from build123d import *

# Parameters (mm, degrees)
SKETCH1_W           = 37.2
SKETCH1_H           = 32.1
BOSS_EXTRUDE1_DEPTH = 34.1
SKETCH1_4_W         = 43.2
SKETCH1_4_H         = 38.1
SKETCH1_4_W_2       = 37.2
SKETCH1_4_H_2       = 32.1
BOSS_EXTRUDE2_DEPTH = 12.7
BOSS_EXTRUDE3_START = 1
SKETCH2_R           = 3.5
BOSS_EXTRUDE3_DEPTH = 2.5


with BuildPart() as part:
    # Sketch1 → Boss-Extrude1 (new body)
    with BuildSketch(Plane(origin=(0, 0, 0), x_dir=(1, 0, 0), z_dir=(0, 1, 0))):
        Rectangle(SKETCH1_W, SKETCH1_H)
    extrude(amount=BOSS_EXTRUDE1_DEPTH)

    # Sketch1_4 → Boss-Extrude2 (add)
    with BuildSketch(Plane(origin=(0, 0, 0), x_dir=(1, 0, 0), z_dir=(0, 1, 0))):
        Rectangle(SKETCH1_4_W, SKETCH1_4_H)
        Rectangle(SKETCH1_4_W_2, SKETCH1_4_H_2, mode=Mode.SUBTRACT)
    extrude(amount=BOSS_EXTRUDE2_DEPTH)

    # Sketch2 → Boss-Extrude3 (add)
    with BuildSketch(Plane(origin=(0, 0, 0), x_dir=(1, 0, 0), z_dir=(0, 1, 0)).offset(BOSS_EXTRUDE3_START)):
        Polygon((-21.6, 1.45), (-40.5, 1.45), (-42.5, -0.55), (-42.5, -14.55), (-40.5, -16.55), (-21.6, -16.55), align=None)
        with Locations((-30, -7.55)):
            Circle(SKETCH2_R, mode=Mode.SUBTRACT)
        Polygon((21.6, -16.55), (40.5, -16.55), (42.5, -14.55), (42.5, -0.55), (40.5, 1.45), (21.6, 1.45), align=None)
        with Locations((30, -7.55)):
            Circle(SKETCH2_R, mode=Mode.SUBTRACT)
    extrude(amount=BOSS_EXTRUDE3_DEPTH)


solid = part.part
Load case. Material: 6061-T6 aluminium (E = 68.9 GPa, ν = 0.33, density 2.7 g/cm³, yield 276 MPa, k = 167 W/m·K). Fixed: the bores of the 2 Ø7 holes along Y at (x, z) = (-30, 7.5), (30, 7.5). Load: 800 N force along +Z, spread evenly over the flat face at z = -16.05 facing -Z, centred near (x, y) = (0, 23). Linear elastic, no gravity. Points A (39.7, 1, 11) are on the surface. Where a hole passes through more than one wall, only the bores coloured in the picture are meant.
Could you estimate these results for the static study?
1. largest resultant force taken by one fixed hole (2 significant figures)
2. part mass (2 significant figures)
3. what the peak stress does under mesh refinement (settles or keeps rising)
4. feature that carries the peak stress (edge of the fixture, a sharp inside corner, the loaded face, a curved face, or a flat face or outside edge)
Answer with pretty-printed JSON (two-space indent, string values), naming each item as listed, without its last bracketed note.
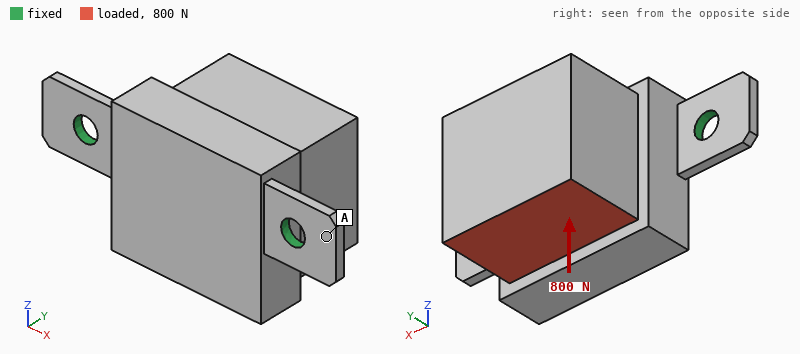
{
  "largest resultant force taken by one fixed hole": "400 N",
  "part mass": "130 g",
  "what the peak stress does under mesh refinement": "keeps rising",
  "feature that carries the peak stress": "edge of the fixture"
}
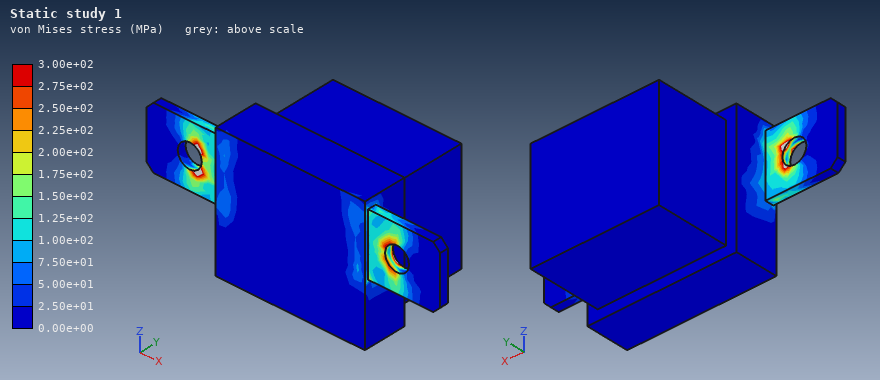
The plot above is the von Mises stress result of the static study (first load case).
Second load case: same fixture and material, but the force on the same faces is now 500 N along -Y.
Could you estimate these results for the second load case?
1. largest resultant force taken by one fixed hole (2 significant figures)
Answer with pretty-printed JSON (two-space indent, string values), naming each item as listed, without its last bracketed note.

{
  "largest resultant force taken by one fixed hole": "270 N"
}
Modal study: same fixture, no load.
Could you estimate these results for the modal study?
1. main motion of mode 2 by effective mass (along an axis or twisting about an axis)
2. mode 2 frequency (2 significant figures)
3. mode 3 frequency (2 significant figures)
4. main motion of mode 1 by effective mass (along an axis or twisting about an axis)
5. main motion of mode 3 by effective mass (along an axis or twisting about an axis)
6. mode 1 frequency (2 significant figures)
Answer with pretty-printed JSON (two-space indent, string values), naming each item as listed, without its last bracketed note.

{
  "main motion of mode 2 by effective mass": "along Y",
  "mode 2 frequency": "4000 Hz",
  "mode 3 frequency": "4400 Hz",
  "main motion of mode 1 by effective mass": "along Z",
  "main motion of mode 3 by effective mass": "along X",
  "mode 1 frequency": "830 Hz"
}
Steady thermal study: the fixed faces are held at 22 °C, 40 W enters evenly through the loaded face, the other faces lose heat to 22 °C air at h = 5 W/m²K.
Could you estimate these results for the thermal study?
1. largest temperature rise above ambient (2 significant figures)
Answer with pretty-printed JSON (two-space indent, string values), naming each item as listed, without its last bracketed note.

{
  "largest temperature rise above ambient": "32 K"
}
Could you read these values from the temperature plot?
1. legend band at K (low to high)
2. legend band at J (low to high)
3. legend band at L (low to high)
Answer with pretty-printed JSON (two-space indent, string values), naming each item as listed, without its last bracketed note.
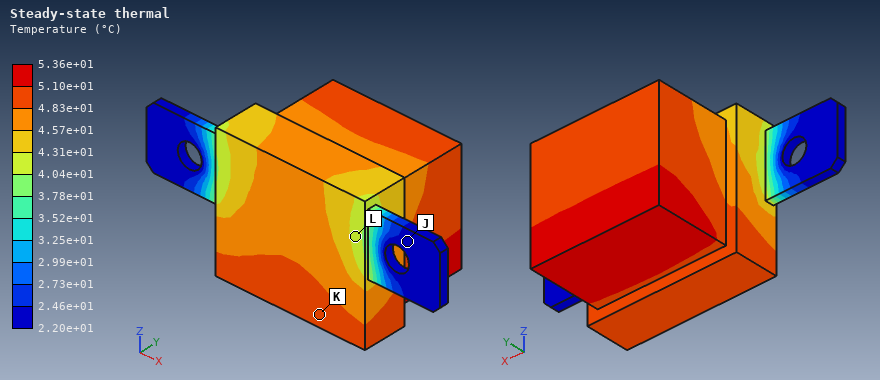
{
  "legend band at K": "4.83e+01 to 5.10e+01 °C",
  "legend band at J": "2.20e+01 to 2.46e+01 °C",
  "legend band at L": "4.04e+01 to 4.31e+01 °C"
}
